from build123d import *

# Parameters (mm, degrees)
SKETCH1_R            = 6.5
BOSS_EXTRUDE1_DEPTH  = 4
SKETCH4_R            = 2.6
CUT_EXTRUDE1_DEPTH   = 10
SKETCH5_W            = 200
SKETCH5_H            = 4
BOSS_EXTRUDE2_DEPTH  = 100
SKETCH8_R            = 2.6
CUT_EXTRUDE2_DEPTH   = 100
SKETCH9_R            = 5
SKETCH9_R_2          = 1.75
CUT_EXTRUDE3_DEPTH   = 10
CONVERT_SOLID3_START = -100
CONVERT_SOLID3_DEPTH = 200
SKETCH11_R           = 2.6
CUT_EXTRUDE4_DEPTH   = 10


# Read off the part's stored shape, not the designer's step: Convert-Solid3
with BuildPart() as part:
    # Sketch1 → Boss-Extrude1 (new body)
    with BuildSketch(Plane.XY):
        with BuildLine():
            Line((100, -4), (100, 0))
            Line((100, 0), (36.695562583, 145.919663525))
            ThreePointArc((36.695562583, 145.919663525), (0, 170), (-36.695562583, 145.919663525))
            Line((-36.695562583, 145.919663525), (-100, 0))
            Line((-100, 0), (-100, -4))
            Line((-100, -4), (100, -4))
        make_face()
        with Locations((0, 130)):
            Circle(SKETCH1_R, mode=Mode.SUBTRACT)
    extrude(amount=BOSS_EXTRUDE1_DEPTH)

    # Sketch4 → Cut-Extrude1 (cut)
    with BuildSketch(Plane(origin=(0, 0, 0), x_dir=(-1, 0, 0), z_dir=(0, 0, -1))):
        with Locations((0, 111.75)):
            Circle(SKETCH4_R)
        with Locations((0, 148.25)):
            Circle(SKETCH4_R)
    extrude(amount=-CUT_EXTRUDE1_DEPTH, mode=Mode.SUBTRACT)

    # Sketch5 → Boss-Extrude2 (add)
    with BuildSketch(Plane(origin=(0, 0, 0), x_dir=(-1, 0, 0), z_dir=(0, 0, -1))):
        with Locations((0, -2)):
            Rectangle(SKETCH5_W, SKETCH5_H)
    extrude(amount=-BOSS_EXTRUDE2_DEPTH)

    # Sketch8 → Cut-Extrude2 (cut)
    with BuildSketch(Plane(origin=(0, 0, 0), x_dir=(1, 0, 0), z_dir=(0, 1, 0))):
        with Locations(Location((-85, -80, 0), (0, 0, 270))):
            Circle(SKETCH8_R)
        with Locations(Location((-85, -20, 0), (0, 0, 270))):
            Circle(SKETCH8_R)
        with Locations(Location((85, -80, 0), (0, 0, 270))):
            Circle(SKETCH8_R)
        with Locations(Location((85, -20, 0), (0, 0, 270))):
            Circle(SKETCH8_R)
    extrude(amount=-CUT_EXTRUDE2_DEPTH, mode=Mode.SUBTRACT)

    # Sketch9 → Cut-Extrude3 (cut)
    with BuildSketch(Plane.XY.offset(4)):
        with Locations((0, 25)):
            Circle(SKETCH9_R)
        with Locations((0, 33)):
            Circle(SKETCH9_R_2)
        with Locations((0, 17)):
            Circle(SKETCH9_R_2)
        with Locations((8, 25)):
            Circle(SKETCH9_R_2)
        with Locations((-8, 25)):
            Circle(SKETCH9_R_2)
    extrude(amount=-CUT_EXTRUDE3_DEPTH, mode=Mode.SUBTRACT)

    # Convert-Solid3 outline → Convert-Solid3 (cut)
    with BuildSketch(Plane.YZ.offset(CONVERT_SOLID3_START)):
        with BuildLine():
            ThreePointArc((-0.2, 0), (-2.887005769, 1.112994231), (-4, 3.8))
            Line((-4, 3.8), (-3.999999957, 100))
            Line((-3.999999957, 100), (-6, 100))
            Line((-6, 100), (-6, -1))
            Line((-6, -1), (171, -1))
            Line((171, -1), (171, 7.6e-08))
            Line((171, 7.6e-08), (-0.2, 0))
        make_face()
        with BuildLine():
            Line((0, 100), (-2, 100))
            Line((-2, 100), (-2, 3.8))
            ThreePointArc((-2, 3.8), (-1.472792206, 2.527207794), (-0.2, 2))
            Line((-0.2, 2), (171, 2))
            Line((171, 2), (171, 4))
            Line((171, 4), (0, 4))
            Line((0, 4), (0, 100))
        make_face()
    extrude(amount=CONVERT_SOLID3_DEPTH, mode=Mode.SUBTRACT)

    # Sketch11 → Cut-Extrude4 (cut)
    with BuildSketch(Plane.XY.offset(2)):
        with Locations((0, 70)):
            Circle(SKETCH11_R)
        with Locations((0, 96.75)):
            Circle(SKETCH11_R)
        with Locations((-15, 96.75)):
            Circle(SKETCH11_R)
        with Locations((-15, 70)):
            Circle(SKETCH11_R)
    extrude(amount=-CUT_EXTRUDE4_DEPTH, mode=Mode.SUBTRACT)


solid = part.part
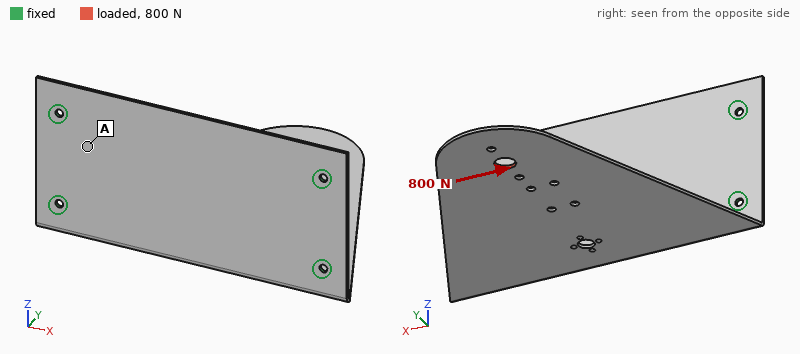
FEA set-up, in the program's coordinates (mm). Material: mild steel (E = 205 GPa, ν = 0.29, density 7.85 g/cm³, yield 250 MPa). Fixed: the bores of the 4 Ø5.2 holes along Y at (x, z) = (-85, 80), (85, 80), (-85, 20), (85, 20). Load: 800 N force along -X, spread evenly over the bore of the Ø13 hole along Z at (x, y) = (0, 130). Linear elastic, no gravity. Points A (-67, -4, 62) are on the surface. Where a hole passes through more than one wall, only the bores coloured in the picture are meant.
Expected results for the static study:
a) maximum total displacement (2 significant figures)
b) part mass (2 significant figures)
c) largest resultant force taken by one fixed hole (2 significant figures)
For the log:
0.51 mm
640 g
750 N
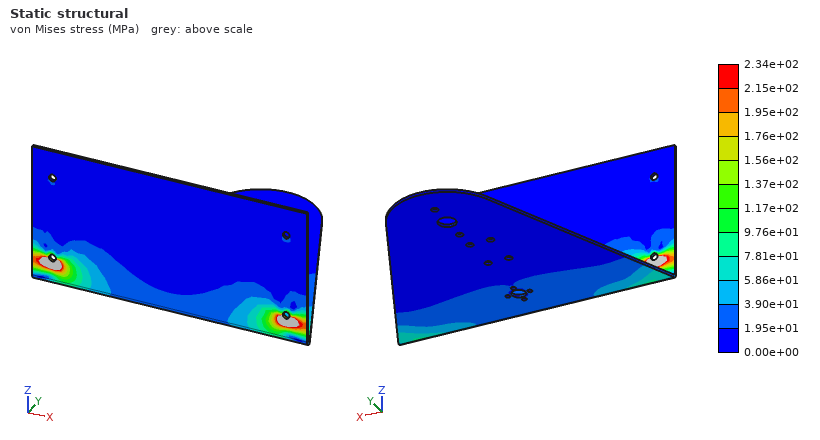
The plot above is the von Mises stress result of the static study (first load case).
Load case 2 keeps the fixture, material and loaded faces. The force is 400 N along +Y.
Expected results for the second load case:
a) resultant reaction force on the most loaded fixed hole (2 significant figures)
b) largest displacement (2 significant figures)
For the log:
240 N
0.62 mm
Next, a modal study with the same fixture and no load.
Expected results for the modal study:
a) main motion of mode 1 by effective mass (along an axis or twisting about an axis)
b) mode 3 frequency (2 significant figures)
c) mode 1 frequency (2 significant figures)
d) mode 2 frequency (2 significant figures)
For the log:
along Z
330 Hz
66 Hz
260 Hz
